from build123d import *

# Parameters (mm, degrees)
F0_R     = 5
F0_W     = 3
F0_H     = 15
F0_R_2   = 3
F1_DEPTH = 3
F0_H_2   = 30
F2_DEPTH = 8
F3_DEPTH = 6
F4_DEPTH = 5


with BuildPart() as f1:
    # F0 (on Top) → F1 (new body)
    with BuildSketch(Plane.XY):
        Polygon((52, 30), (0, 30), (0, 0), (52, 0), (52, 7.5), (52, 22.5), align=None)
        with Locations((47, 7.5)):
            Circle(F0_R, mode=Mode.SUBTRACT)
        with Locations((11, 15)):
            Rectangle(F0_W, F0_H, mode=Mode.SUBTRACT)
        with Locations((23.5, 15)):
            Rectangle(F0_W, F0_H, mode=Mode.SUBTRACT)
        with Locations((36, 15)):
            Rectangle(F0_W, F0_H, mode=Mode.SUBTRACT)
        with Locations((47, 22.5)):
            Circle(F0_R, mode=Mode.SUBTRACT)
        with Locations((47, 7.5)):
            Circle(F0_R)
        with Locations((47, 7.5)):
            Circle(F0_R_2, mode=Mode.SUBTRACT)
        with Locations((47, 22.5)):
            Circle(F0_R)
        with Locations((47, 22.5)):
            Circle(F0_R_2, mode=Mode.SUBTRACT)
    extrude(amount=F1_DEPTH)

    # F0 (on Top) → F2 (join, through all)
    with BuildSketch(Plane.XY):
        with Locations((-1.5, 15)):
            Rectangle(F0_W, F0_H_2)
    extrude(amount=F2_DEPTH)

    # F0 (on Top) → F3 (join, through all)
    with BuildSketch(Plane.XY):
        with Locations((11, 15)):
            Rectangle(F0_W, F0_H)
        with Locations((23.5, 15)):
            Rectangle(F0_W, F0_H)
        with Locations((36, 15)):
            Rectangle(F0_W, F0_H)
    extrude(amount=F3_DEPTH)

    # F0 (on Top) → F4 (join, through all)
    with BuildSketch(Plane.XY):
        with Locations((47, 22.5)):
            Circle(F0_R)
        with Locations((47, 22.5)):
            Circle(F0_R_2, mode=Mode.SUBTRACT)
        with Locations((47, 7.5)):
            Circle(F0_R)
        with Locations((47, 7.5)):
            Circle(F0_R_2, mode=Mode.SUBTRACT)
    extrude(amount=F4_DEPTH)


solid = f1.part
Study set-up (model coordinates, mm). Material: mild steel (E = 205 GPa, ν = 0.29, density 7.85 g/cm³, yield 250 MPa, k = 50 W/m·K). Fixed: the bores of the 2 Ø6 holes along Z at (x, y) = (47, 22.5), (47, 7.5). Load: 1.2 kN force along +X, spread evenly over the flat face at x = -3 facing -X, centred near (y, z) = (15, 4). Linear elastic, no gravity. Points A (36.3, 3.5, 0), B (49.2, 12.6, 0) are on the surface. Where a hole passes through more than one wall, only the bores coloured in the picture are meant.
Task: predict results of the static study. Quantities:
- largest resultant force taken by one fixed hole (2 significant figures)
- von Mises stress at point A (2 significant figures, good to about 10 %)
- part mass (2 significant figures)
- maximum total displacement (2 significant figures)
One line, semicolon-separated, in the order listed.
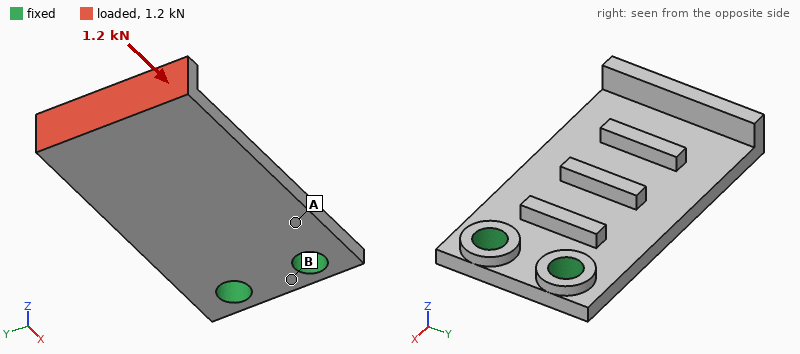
600 N; 48 MPa; 46 g; 0.23 mm
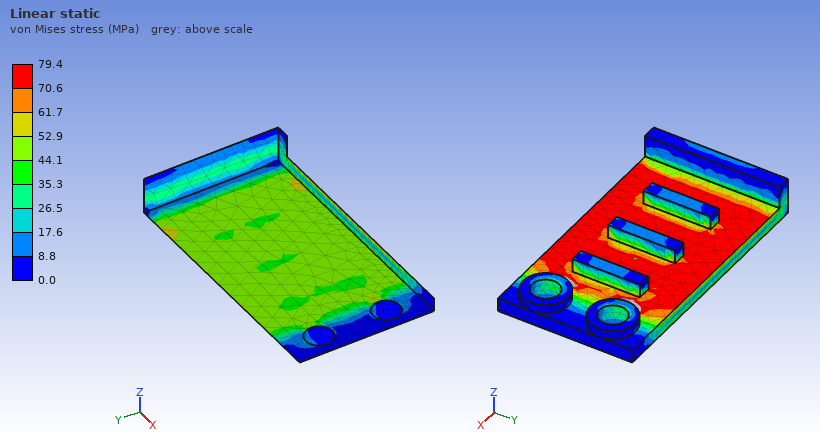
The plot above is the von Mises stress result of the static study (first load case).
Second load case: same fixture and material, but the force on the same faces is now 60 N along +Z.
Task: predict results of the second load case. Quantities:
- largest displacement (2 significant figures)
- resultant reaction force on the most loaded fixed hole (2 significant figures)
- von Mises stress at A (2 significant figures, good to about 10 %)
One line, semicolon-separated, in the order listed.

0.14 mm; 30 N; 48 MPa
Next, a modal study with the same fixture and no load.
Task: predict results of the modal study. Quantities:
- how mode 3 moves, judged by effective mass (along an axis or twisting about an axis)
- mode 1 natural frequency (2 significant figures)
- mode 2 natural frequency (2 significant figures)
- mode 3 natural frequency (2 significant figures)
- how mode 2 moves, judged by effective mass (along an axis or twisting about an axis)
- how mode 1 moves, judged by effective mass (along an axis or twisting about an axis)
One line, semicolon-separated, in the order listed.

along Z; 960 Hz; 3500 Hz; 5900 Hz; twisting about X; along Z
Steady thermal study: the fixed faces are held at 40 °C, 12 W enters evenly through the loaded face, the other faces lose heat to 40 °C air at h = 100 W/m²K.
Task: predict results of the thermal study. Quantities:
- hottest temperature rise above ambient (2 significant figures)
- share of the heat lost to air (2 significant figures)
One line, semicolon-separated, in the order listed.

60 K; 74 %
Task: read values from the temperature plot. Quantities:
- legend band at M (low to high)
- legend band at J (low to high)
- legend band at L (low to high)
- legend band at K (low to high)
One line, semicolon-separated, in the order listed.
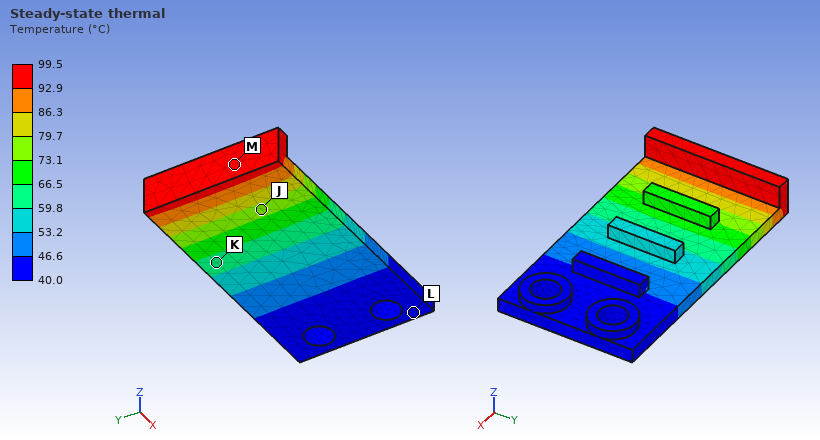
92.9 to 99.5 °C; 73.1 to 79.7 °C; 40.0 to 46.6 °C; 59.8 to 66.5 °C
